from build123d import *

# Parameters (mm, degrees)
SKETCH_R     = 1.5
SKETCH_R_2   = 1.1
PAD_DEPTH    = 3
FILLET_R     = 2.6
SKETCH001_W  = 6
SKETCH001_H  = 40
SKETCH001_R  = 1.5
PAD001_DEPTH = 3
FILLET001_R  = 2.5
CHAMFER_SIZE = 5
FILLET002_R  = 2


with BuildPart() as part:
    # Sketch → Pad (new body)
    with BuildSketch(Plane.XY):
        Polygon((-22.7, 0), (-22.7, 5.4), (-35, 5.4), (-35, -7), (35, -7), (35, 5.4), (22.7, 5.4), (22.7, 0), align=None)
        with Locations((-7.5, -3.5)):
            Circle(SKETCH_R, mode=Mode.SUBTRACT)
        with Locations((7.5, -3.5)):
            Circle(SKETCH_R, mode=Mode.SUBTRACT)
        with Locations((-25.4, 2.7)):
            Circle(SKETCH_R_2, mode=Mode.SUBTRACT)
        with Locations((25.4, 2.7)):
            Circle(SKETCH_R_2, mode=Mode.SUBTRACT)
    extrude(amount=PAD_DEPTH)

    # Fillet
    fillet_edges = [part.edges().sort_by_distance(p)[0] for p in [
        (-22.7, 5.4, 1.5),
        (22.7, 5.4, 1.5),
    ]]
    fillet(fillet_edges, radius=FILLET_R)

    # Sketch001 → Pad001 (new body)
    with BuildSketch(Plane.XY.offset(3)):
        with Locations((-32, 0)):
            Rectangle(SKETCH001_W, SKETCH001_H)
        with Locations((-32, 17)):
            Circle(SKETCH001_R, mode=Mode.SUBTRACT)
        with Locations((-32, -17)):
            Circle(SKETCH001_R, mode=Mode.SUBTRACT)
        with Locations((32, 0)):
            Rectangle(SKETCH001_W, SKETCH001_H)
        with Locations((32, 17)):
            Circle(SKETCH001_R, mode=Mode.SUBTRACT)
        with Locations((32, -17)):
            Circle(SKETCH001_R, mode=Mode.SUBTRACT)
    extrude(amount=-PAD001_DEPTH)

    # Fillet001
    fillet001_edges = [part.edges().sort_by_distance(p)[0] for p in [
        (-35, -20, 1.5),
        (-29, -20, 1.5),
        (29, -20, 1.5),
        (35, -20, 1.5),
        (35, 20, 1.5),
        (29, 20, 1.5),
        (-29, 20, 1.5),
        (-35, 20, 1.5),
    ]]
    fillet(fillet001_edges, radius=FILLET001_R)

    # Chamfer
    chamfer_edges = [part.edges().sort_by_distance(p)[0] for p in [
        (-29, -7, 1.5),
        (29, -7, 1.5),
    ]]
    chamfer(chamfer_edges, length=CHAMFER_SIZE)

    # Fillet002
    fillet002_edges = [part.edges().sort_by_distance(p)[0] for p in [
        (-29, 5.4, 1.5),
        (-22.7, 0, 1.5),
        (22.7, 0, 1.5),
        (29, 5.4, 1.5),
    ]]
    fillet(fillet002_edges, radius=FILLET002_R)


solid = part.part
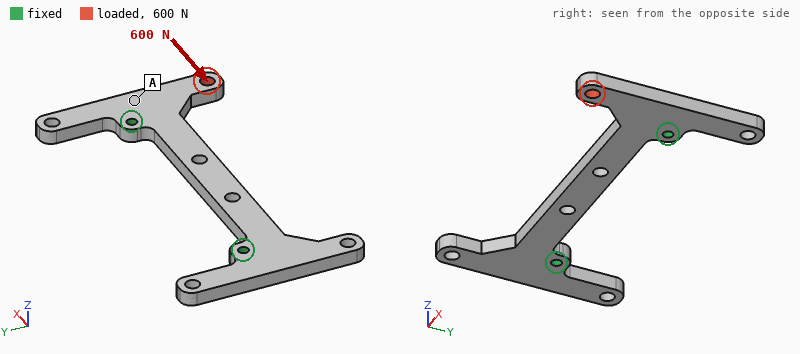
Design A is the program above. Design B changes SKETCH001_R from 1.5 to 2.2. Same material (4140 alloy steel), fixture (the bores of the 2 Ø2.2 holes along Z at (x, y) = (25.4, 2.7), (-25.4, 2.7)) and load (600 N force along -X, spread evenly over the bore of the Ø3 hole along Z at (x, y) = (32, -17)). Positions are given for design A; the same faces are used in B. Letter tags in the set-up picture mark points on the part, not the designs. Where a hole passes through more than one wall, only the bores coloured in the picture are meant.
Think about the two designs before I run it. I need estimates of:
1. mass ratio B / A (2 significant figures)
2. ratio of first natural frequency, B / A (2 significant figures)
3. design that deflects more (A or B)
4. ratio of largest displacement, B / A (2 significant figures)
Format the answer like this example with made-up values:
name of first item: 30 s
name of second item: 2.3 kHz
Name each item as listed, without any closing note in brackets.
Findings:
mass ratio B / A: 0.96
ratio of first natural frequency, B / A: 1.0
design that deflects more: B
ratio of largest displacement, B / A: 1.2
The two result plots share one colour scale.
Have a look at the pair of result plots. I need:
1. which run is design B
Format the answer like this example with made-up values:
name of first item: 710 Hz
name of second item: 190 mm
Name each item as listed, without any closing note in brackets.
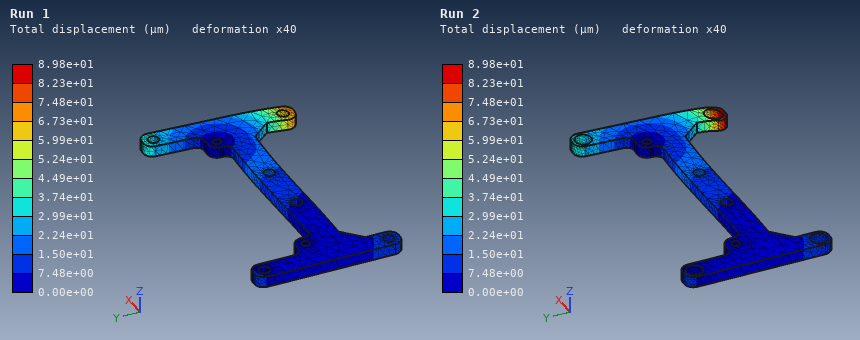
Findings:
which run is design B: Run 2
